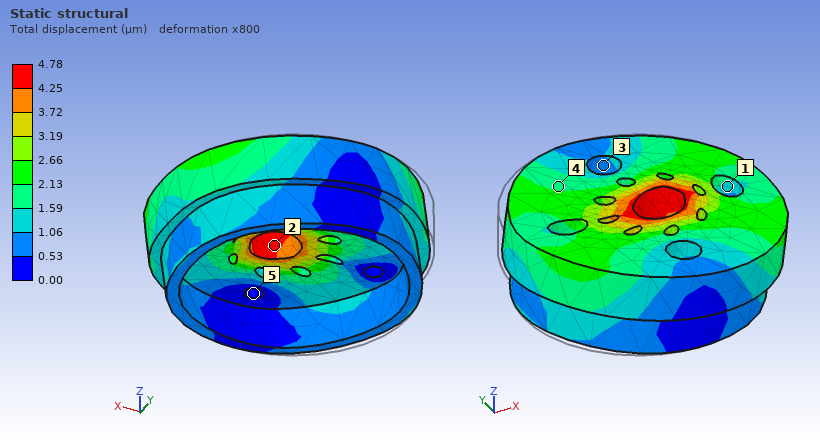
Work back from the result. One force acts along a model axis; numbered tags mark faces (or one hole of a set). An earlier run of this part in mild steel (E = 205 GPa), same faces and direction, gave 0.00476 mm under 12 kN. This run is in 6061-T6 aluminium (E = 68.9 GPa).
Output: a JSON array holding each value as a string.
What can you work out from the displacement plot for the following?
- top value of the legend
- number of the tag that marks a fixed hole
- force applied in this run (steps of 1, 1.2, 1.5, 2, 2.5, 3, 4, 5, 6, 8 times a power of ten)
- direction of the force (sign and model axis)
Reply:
["4.78 µm", "5", "4 kN", "+X"]
